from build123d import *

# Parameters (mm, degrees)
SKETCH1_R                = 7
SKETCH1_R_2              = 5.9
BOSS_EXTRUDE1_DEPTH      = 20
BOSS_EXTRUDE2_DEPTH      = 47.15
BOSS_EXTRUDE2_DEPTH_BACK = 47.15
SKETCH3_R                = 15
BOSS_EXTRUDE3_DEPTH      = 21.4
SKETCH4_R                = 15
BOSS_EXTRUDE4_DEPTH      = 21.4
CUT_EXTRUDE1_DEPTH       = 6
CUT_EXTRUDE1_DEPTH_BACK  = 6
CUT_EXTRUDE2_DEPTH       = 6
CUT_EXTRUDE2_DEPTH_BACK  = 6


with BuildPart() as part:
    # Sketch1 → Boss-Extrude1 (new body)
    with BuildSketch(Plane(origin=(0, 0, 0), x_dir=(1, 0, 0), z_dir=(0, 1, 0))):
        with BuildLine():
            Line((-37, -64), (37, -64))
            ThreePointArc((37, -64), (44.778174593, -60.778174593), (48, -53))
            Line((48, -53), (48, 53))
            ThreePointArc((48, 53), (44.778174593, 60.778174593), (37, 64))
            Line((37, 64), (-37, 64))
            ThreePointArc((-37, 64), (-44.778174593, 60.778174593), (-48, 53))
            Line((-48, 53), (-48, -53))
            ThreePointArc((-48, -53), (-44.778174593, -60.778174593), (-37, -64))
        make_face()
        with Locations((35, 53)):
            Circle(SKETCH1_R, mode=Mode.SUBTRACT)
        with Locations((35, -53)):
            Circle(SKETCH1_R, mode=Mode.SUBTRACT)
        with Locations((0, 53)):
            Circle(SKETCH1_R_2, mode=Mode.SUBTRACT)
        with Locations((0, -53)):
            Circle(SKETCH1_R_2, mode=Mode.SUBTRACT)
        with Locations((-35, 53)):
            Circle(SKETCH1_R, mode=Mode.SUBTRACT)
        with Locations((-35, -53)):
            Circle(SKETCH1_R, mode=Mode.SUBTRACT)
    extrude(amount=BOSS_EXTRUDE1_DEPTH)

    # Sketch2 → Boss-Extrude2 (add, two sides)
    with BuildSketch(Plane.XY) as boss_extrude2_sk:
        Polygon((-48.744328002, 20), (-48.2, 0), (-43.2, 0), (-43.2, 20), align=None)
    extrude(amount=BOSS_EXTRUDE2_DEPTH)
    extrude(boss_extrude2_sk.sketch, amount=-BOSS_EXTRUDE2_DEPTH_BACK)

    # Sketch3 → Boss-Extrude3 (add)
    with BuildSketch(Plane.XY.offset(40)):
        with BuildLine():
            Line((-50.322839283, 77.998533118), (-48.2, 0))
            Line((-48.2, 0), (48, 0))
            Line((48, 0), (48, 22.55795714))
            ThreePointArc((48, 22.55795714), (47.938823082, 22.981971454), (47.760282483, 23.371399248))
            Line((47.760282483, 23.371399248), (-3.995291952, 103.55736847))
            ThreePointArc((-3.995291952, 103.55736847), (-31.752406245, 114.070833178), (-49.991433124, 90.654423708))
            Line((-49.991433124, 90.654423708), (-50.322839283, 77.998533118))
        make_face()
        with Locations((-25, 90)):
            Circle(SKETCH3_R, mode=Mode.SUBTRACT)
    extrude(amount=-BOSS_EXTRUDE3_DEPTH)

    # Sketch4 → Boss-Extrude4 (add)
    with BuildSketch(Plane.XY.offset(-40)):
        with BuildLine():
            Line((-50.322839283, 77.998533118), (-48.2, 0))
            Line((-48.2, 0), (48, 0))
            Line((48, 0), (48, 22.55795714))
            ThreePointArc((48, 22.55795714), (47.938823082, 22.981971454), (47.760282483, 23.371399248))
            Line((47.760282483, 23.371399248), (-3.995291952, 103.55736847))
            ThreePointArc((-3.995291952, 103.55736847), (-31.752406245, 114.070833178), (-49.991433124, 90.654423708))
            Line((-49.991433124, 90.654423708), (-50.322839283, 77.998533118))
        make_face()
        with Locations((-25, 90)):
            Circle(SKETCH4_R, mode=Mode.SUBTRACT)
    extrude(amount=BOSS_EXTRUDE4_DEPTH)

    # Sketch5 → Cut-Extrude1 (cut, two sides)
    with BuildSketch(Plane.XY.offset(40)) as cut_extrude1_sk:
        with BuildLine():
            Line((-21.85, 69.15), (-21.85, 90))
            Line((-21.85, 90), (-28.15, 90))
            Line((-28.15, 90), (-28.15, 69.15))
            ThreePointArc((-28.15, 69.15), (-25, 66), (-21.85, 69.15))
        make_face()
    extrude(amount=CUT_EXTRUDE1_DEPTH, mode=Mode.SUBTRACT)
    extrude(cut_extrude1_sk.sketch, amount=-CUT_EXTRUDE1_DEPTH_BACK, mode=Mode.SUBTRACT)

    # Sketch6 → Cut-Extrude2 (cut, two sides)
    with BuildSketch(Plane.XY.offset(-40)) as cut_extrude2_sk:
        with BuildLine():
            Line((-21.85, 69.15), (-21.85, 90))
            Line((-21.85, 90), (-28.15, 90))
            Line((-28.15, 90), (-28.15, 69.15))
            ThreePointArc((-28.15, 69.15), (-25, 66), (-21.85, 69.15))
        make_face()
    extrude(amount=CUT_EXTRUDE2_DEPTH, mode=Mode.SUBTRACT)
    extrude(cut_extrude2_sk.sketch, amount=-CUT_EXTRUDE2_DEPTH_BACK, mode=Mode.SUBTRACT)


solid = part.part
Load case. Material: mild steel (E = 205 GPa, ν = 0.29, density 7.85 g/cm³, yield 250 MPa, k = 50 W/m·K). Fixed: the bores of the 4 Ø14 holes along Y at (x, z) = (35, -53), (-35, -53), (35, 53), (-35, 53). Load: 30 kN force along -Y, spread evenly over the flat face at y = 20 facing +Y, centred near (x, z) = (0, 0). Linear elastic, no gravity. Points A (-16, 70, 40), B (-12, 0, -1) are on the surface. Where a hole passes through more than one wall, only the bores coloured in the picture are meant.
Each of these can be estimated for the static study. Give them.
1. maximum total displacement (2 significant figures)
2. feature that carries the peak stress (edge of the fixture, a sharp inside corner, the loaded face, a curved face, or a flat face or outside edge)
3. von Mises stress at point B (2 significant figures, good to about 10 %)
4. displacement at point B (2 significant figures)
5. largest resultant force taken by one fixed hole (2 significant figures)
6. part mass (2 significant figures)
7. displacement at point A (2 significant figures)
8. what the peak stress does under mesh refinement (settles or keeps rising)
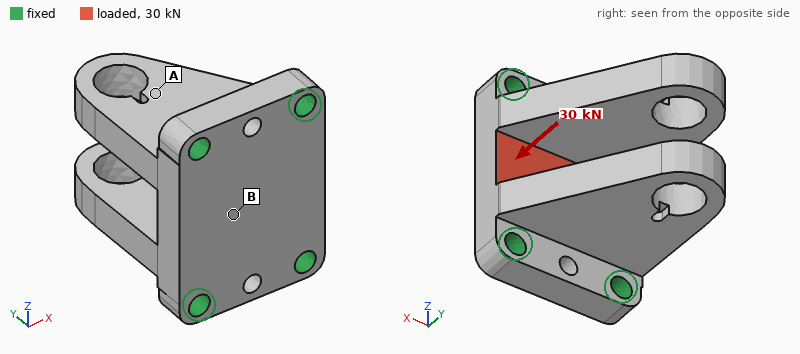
46 µm
edge of the fixture
38 MPa
17 µm
7.6 kN
3.7 kg
25 µm
keeps rising
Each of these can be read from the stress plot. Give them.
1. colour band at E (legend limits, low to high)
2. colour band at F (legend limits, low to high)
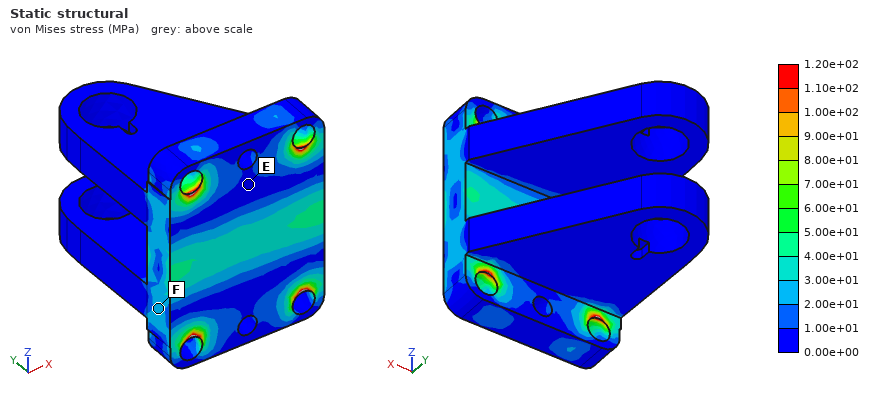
0.00e+00 to 1.00e+01 MPa
2.00e+01 to 3.00e+01 MPa
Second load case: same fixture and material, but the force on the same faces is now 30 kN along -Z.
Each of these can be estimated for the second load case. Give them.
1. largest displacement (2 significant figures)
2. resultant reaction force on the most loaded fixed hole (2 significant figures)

3.1 µm
7.9 kN
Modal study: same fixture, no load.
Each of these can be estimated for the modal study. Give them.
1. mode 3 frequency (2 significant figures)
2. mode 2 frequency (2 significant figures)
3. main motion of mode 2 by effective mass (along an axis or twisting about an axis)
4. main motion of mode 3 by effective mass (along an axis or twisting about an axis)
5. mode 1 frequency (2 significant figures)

4400 Hz
2400 Hz
along Z
along X
2000 Hz
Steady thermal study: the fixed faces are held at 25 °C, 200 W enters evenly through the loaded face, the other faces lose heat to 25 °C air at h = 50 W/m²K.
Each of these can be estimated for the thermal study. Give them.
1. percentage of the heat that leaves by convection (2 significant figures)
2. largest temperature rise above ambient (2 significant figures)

23 %
44 K
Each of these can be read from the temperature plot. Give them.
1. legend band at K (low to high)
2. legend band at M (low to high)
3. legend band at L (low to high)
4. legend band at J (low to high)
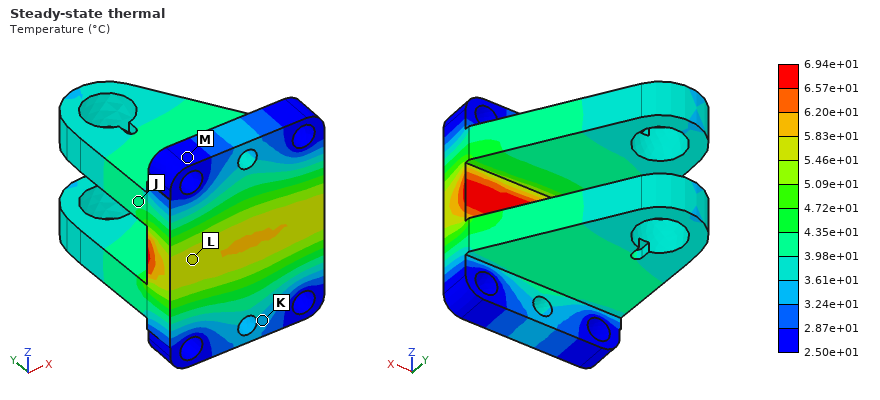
3.24e+01 to 3.61e+01 °C
2.50e+01 to 2.87e+01 °C
5.46e+01 to 5.83e+01 °C
3.98e+01 to 4.35e+01 °C
